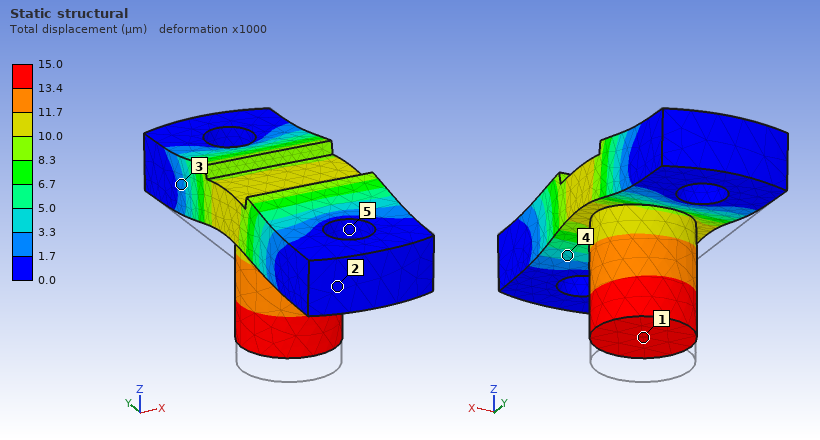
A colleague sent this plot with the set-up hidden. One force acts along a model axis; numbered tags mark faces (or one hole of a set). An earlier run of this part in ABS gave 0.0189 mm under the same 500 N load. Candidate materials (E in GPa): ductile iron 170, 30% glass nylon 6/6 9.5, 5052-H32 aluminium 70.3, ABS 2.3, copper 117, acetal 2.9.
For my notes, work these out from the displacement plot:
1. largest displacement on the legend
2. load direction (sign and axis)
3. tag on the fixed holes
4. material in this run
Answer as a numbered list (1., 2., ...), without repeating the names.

1. 15.0 µm
2. +Z
3. 5
4. acetal
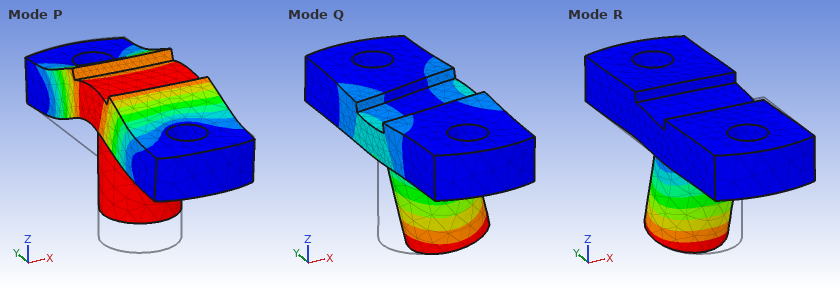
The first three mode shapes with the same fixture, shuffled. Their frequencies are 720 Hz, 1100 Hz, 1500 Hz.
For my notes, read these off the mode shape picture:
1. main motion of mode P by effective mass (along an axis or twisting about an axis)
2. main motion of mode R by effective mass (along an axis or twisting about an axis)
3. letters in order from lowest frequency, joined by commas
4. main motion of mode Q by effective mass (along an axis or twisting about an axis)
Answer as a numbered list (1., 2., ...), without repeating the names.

1. along Z
2. along Y
3. Q, R, P
4. along X
